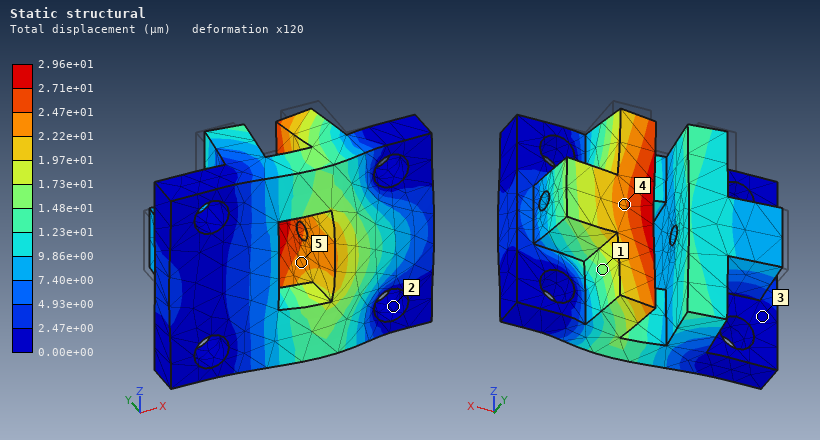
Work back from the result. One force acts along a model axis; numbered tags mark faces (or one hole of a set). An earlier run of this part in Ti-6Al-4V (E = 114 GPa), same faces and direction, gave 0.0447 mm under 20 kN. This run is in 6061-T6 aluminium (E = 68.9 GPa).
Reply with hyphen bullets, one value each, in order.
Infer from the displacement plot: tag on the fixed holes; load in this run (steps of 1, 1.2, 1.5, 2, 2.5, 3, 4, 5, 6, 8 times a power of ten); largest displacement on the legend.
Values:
- 2
- 8 kN
- 2.96e+01 µm
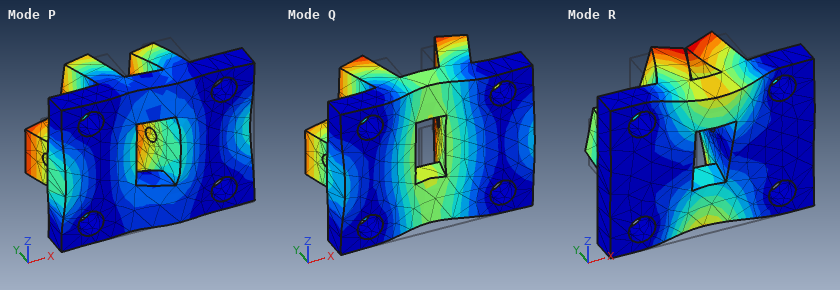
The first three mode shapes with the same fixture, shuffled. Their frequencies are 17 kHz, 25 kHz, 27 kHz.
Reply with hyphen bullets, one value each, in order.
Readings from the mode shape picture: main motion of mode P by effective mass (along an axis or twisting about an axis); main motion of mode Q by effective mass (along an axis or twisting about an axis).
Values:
- along X
- along Y
